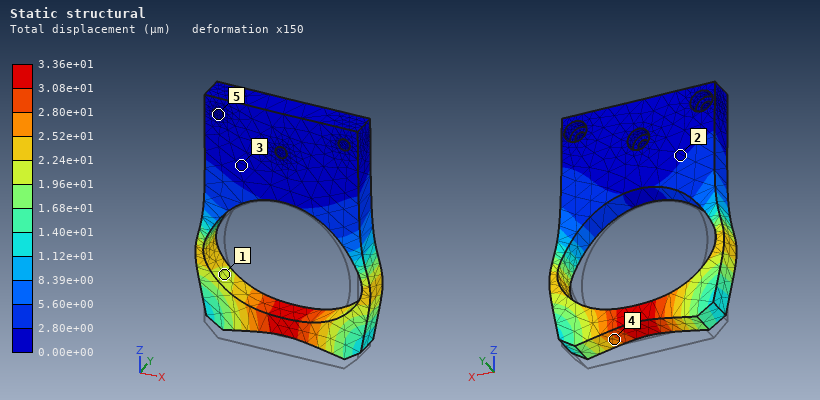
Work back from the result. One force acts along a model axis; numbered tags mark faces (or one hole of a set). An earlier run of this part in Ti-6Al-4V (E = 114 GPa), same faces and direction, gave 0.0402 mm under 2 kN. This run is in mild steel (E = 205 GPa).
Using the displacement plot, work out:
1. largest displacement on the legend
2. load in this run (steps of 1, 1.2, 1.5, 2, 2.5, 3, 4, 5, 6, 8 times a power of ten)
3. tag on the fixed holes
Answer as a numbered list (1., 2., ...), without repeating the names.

1. 3.36e+01 µm
2. 3 kN
3. 5
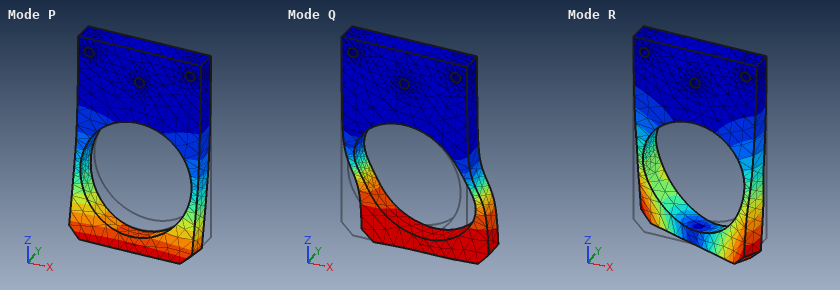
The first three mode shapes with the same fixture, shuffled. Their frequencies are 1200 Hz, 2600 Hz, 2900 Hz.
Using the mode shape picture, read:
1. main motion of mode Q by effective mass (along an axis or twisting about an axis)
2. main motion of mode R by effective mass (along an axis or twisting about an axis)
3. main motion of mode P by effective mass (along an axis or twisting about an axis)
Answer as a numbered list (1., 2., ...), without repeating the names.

1. along X
2. twisting about Z
3. along Y
